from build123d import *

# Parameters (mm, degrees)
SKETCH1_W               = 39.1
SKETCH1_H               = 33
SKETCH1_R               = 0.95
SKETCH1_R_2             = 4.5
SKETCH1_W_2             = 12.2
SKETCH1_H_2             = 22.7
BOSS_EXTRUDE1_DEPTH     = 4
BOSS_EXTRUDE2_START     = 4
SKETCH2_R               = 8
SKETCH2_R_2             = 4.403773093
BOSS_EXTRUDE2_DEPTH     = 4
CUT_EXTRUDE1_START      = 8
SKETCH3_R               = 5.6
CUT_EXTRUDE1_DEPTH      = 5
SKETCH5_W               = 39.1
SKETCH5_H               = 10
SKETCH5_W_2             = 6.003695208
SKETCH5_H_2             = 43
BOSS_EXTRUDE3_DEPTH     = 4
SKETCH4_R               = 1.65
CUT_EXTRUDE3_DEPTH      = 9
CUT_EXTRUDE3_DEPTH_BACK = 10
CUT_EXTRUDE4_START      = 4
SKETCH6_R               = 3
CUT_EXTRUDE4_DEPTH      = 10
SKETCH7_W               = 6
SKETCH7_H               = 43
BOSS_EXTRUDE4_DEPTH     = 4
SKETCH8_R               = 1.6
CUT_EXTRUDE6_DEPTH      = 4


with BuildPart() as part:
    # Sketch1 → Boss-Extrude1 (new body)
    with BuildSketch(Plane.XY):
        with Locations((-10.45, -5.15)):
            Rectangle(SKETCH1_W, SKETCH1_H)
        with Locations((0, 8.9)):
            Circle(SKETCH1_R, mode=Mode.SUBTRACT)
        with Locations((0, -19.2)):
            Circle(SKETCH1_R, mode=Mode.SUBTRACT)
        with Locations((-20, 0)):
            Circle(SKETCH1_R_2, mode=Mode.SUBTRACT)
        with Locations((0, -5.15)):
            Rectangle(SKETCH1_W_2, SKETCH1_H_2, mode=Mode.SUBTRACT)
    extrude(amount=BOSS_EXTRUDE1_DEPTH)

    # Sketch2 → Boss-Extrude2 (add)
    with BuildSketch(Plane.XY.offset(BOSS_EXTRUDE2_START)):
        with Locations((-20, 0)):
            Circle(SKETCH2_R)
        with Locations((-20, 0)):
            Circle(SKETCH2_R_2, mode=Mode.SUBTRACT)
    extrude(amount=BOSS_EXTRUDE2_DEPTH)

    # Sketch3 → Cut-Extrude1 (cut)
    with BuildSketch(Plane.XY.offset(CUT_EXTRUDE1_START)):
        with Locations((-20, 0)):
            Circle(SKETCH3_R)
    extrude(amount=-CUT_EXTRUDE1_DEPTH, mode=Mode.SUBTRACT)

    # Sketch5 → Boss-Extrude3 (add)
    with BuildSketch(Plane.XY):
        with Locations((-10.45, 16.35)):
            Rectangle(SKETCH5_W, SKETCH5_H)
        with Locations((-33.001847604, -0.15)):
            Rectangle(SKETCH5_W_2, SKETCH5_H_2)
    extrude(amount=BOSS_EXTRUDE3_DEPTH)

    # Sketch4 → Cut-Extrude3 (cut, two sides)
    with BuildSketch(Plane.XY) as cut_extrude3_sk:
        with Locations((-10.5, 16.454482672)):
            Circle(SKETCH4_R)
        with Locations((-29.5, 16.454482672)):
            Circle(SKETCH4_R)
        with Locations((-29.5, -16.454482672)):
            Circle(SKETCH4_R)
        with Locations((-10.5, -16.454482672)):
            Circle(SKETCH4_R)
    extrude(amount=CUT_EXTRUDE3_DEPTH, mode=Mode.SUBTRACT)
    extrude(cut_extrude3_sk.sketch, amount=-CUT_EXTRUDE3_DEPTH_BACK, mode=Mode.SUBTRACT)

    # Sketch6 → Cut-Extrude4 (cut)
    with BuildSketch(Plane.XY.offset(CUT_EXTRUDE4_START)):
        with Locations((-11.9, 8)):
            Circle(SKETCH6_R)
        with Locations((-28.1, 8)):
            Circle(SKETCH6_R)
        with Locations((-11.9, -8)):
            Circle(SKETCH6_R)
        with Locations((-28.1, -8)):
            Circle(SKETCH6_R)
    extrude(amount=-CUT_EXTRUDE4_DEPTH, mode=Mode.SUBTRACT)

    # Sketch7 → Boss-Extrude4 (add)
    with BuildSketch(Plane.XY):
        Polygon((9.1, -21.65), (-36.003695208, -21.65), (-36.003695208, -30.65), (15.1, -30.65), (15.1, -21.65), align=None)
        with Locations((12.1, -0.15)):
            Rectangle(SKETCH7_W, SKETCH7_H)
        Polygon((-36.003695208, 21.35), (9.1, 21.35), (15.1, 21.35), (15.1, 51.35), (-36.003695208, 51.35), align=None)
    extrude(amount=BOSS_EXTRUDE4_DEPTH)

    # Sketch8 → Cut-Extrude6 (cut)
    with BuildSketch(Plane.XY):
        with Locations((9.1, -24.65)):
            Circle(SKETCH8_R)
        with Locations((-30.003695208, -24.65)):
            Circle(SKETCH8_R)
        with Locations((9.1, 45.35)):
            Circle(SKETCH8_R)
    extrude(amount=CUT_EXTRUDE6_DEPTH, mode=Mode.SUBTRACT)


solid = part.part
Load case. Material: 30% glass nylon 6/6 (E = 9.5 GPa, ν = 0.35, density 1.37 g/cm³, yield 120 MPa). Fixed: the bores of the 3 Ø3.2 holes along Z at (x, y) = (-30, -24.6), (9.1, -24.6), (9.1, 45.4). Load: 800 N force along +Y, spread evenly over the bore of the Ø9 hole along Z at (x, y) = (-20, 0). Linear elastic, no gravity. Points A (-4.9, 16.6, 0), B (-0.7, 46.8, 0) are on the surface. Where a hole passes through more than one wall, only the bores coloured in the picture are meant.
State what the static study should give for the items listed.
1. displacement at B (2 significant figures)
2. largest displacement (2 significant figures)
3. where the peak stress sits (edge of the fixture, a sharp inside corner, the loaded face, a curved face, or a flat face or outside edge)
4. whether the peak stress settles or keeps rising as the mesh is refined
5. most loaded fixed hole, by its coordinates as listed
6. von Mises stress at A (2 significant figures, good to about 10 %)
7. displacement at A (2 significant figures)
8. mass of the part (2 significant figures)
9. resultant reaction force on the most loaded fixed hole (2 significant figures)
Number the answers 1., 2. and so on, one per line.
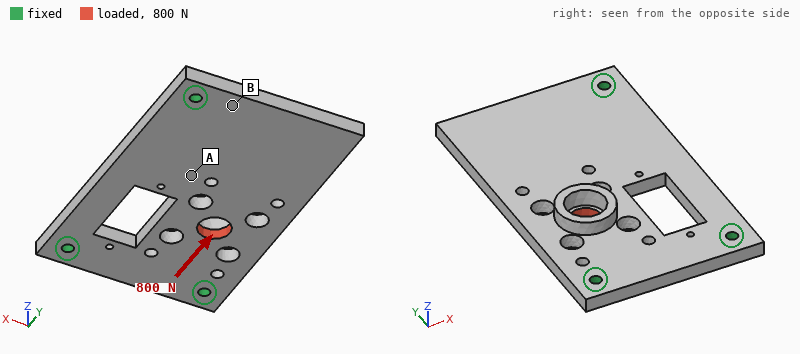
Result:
1. 11 µm
2. 67 µm
3. edge of the fixture
4. keeps rising
5. (-30, -24.6)
6. 4.1 MPa
7. 30 µm
8. 21 g
9. 460 N
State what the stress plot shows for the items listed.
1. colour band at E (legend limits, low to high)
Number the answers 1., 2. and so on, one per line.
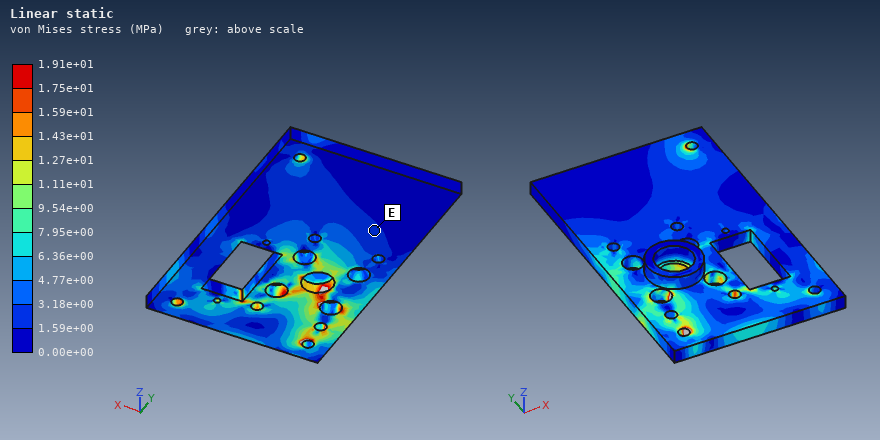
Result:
1. 1.59e+00 to 3.18e+00 MPa
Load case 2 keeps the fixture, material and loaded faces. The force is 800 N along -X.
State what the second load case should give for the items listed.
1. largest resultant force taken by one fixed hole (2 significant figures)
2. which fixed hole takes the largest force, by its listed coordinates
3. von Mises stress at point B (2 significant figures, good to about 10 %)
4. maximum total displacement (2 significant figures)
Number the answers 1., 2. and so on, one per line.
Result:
1. 330 N
2. (9.1, 45.4)
3. 4.3 MPa
4. 77 µm
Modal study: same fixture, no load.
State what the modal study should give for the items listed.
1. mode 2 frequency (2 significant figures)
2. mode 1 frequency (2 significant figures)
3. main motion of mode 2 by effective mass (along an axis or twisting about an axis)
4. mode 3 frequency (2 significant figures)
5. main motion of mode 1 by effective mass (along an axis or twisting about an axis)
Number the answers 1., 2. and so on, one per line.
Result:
1. 1900 Hz
2. 920 Hz
3. along Z
4. 2900 Hz
5. along Z
